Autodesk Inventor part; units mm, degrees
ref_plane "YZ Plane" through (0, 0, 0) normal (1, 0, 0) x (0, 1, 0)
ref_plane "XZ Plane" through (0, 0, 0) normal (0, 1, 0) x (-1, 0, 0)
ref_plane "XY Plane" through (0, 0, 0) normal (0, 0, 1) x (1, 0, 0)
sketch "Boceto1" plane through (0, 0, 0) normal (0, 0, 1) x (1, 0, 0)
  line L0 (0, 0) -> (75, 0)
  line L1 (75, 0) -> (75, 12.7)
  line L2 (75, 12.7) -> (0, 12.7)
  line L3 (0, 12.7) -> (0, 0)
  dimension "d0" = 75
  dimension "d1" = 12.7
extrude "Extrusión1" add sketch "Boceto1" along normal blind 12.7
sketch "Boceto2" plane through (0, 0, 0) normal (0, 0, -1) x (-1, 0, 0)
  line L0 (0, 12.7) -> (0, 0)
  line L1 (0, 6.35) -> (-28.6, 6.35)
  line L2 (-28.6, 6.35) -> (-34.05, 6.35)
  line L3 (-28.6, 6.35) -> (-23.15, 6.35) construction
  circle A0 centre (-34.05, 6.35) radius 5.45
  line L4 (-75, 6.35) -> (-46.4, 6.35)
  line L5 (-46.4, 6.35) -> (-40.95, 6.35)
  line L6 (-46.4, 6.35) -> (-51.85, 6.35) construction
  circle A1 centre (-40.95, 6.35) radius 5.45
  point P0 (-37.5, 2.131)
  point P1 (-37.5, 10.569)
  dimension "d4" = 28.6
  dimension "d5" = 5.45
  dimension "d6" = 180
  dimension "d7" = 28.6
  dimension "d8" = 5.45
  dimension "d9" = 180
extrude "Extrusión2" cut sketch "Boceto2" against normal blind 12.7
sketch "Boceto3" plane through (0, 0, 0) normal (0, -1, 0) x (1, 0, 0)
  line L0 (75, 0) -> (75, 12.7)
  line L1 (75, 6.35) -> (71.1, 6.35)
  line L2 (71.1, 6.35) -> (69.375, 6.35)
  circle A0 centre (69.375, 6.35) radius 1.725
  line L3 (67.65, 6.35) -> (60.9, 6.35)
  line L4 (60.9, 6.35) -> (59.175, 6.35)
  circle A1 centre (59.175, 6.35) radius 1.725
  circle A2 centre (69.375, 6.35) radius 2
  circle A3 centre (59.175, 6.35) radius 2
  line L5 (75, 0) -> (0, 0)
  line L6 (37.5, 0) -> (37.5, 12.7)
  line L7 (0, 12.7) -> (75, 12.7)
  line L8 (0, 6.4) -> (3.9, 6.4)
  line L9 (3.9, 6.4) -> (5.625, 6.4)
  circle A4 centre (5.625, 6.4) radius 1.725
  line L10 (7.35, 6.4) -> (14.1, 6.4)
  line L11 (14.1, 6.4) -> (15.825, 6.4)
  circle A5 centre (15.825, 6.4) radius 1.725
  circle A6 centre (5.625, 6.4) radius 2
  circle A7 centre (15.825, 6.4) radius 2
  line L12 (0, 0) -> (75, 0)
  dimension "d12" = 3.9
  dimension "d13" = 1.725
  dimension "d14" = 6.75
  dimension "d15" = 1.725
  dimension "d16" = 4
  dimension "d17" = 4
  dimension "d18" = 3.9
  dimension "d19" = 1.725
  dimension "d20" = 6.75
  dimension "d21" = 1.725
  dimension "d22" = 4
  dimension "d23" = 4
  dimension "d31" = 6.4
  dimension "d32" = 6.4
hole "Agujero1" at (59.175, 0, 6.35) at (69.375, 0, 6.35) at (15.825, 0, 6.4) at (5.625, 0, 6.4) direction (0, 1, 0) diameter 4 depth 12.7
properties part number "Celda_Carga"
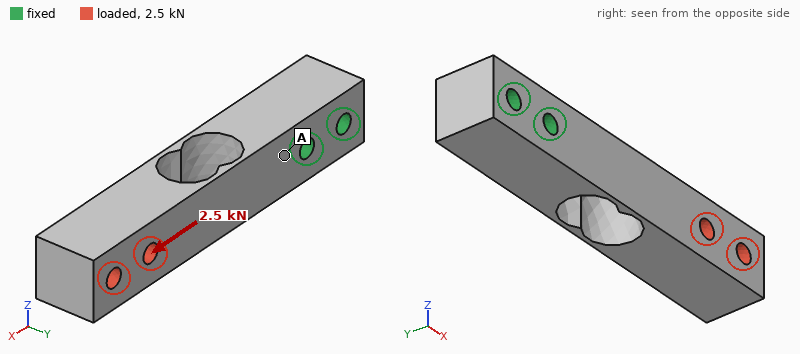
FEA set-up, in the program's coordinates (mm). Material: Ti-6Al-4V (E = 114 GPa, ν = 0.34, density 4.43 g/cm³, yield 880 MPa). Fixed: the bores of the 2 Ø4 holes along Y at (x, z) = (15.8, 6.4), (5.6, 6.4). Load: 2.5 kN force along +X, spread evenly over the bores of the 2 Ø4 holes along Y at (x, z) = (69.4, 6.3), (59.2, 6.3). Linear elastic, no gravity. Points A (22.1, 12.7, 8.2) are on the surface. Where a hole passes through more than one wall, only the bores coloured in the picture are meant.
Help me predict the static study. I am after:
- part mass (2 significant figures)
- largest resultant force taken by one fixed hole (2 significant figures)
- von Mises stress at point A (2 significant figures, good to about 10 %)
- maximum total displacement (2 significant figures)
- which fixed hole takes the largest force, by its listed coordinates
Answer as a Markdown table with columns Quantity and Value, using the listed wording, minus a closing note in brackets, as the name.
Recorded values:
| Quantity | Value |
|---|---|
| part mass | 42 g |
| largest resultant force taken by one fixed hole | 2.2 kN |
| von Mises stress at point A | 27 MPa |
| maximum total displacement | 21 µm |
| which fixed hole takes the largest force, by its listed coordinates | (15.8, 6.4) |
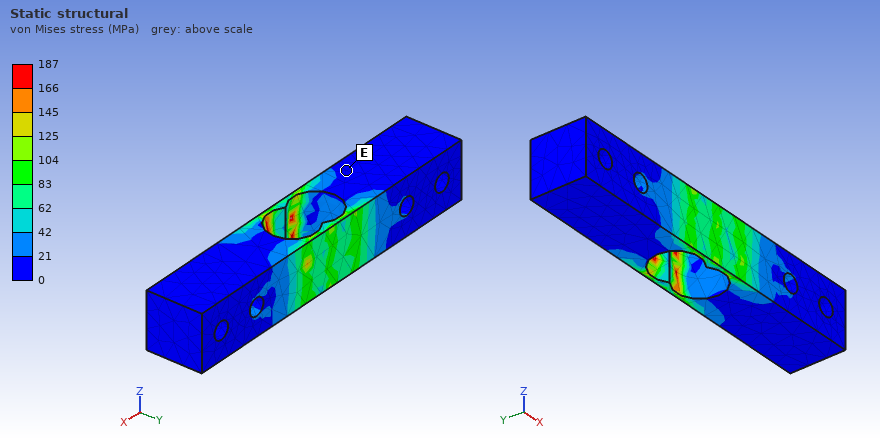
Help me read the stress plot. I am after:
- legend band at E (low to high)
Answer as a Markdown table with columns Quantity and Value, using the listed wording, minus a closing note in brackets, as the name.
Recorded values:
| Quantity | Value |
|---|---|
| legend band at E | 0 to 21 MPa |
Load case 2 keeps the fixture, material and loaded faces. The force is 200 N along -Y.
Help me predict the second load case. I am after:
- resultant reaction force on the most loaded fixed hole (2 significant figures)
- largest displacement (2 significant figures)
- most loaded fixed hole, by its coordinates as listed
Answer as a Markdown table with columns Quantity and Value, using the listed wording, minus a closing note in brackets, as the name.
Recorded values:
| Quantity | Value |
|---|---|
| resultant reaction force on the most loaded fixed hole | 310 N |
| largest displacement | 0.17 mm |
| most loaded fixed hole, by its coordinates as listed | (15.8, 6.4) |
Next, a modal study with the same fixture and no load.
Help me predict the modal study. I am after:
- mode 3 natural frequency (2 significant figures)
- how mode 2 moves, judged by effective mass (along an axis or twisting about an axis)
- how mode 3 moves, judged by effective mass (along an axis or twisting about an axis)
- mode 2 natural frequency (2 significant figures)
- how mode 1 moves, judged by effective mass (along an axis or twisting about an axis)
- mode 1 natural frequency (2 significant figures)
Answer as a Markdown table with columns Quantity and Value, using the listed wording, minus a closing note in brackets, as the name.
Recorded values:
| Quantity | Value |
|---|---|
| mode 3 natural frequency | 6500 Hz |
| how mode 2 moves, judged by effective mass | along Z |
| how mode 3 moves, judged by effective mass | twisting about X |
| mode 2 natural frequency | 1800 Hz |
| how mode 1 moves, judged by effective mass | along Y |
| mode 1 natural frequency | 1300 Hz |
